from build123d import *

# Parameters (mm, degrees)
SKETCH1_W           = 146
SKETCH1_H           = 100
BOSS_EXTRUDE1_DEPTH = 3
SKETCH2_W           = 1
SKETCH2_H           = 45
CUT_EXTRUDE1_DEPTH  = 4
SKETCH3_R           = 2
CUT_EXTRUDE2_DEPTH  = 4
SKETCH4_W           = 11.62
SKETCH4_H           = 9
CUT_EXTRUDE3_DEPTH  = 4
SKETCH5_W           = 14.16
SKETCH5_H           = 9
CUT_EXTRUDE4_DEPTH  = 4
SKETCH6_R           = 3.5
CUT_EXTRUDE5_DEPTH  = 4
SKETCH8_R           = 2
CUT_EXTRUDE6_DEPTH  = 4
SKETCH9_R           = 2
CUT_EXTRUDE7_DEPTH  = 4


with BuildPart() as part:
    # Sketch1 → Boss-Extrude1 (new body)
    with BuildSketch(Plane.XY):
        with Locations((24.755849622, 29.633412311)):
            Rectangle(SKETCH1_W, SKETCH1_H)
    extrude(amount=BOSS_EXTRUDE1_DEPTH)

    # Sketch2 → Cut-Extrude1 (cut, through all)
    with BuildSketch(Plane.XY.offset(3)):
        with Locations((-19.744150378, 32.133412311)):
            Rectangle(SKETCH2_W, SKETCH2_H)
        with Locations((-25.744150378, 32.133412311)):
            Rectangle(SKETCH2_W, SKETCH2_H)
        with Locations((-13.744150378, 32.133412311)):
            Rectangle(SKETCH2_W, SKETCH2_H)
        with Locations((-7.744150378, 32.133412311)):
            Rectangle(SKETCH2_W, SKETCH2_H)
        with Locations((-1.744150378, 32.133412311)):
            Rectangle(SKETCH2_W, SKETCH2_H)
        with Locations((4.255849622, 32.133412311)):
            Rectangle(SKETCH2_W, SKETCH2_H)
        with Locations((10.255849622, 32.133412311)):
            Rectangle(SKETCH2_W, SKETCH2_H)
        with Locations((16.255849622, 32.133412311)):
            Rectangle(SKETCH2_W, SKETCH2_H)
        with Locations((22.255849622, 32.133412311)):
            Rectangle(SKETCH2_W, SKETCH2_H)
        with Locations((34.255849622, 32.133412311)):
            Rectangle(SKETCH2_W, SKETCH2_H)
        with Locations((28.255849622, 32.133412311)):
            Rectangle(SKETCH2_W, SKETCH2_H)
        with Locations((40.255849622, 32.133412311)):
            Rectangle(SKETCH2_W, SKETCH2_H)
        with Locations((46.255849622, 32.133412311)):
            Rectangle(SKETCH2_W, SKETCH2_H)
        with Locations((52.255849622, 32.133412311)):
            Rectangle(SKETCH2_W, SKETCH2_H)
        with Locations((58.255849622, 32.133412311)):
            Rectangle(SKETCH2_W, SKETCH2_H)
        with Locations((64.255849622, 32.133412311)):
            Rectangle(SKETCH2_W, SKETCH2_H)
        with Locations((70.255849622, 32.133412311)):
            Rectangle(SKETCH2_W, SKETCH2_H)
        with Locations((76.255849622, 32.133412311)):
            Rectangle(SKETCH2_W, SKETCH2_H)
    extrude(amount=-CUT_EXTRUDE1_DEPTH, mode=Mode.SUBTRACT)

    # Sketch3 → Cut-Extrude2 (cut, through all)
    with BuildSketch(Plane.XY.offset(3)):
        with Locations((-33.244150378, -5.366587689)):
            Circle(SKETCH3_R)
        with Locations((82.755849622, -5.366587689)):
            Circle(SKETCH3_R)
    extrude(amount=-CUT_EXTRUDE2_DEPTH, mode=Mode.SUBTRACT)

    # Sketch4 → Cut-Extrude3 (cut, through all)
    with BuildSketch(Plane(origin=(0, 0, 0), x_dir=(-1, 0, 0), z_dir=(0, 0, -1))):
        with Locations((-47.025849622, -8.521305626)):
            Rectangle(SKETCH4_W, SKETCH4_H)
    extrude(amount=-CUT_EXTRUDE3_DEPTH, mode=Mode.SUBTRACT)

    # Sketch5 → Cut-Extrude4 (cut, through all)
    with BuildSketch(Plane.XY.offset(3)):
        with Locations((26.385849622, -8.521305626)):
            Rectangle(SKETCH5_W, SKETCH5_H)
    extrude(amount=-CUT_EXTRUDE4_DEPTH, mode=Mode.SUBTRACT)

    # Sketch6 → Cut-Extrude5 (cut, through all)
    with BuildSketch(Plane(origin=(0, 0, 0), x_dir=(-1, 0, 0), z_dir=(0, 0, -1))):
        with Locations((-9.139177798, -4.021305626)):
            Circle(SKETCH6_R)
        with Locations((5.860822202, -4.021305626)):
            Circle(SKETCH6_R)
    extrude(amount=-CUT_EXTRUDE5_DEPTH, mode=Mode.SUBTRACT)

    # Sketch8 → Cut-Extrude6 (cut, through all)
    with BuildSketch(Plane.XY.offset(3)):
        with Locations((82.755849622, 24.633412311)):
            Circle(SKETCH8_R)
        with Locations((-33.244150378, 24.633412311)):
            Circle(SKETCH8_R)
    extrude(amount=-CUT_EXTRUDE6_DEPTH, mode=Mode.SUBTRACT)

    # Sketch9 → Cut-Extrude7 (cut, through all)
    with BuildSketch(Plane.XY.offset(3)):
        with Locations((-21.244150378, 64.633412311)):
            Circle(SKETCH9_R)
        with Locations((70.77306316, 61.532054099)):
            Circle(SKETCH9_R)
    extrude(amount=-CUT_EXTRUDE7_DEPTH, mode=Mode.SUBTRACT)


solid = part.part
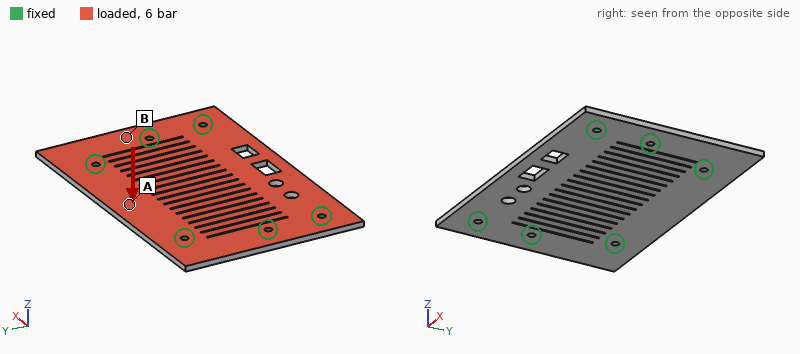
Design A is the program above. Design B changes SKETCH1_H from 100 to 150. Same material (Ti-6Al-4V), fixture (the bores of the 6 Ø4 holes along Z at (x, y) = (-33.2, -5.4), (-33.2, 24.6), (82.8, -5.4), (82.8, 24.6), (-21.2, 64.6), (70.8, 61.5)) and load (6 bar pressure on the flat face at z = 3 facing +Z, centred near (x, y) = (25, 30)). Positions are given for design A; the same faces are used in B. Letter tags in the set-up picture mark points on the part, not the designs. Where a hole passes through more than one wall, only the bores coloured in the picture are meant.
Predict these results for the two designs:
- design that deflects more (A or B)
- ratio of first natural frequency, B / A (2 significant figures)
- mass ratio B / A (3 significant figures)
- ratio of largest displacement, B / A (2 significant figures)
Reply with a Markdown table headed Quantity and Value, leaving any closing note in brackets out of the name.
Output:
| Quantity | Value |
|---|---|
| design that deflects more | B |
| ratio of first natural frequency, B / A | 0.82 |
| mass ratio B / A | 1.54 |
| ratio of largest displacement, B / A | 1.8 |
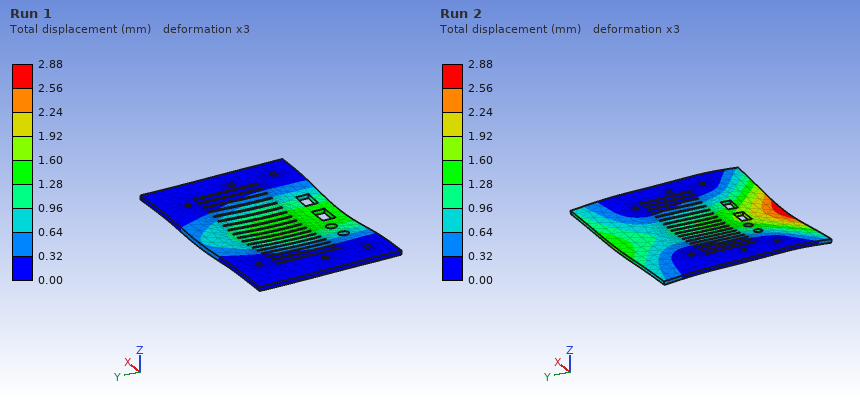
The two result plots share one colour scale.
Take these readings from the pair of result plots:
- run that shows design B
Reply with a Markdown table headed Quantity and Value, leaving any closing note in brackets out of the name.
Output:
| Quantity | Value |
|---|---|
| run that shows design B | Run 2 |
